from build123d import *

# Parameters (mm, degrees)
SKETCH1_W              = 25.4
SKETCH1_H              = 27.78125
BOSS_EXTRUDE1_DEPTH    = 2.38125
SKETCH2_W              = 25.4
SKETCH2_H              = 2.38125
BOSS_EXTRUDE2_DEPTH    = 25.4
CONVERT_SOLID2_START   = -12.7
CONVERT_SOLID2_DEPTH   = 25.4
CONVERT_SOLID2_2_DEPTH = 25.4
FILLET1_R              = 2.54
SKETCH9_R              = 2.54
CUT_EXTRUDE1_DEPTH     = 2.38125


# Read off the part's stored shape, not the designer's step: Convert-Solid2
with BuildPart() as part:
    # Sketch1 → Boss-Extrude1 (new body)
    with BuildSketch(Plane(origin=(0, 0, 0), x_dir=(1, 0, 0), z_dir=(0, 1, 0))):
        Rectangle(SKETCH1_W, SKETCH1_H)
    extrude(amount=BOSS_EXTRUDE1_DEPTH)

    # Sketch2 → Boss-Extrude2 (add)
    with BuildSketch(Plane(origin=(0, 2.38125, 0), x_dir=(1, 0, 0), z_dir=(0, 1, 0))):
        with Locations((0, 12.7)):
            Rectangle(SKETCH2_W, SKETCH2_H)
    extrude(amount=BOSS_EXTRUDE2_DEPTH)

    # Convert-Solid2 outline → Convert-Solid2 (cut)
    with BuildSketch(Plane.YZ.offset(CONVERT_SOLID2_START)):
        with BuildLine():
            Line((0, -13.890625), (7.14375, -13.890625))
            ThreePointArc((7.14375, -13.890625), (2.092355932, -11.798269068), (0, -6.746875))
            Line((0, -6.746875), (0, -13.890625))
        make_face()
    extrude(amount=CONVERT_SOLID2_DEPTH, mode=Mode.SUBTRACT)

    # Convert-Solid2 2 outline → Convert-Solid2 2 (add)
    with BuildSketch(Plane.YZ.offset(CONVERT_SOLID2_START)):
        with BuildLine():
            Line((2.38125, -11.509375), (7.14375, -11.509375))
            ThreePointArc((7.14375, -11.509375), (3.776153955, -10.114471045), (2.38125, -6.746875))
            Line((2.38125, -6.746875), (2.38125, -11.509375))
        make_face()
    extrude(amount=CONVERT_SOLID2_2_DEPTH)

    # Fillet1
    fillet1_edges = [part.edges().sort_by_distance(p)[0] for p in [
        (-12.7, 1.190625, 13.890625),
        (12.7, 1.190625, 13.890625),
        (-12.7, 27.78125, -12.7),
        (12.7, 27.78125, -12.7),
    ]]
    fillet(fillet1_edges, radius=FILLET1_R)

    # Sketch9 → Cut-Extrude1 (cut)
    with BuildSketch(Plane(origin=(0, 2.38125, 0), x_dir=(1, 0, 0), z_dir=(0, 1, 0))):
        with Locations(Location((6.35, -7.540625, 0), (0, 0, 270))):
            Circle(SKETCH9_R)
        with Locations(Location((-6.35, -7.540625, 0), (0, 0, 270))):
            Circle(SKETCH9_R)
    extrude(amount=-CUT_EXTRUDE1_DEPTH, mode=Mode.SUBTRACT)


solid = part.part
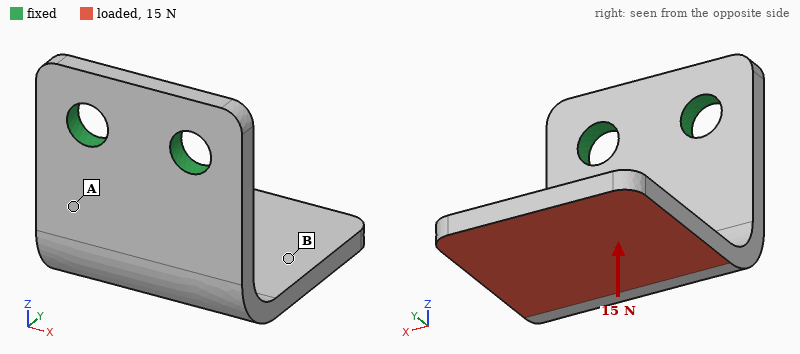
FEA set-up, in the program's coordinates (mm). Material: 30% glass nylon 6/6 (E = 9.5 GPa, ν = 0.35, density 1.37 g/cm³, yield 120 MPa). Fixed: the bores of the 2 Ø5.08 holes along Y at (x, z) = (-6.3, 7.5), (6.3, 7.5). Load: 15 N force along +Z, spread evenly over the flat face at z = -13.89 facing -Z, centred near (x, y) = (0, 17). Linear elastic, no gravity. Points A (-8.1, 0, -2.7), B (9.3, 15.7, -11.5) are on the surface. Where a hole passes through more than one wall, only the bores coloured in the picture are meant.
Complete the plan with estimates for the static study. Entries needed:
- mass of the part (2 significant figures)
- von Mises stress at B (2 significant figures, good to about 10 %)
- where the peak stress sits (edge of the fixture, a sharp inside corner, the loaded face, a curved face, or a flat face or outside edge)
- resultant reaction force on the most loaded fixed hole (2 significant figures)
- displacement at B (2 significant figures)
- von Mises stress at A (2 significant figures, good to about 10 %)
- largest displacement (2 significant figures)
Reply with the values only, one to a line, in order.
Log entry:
4.0 g
2.1 MPa
a flat face or outside edge
8.0 N
0.28 mm
9.0 MPa
0.53 mm
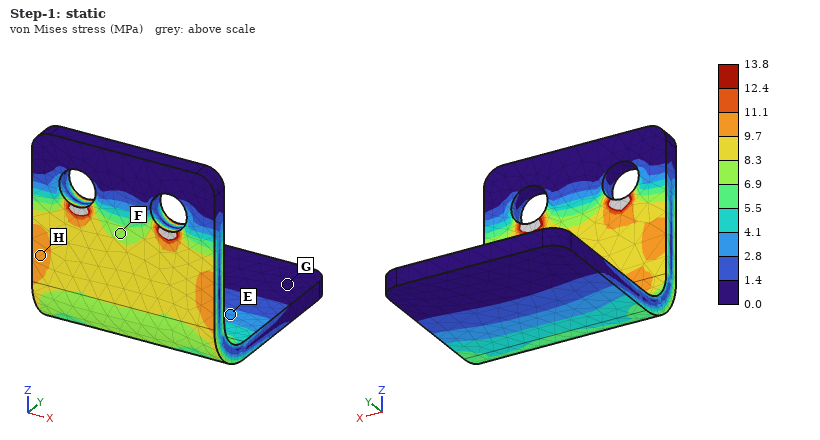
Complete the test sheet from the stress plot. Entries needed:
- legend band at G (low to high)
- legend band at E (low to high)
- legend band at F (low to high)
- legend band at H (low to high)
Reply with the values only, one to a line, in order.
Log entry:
0.0 to 1.4 MPa
2.8 to 4.1 MPa
6.9 to 8.3 MPa
9.7 to 11.1 MPa
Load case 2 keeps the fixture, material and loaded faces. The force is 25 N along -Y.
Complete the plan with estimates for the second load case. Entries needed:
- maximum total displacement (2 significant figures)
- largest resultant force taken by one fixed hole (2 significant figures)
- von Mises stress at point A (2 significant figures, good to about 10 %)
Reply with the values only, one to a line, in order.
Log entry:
0.52 mm
13 N
11 MPa
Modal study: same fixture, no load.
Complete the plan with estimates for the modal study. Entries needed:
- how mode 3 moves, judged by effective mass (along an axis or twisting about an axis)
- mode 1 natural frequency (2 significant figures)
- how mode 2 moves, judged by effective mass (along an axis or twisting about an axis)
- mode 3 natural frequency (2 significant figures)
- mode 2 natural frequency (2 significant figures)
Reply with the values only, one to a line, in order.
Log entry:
along Y
710 Hz
along X
2200 Hz
1200 Hz
